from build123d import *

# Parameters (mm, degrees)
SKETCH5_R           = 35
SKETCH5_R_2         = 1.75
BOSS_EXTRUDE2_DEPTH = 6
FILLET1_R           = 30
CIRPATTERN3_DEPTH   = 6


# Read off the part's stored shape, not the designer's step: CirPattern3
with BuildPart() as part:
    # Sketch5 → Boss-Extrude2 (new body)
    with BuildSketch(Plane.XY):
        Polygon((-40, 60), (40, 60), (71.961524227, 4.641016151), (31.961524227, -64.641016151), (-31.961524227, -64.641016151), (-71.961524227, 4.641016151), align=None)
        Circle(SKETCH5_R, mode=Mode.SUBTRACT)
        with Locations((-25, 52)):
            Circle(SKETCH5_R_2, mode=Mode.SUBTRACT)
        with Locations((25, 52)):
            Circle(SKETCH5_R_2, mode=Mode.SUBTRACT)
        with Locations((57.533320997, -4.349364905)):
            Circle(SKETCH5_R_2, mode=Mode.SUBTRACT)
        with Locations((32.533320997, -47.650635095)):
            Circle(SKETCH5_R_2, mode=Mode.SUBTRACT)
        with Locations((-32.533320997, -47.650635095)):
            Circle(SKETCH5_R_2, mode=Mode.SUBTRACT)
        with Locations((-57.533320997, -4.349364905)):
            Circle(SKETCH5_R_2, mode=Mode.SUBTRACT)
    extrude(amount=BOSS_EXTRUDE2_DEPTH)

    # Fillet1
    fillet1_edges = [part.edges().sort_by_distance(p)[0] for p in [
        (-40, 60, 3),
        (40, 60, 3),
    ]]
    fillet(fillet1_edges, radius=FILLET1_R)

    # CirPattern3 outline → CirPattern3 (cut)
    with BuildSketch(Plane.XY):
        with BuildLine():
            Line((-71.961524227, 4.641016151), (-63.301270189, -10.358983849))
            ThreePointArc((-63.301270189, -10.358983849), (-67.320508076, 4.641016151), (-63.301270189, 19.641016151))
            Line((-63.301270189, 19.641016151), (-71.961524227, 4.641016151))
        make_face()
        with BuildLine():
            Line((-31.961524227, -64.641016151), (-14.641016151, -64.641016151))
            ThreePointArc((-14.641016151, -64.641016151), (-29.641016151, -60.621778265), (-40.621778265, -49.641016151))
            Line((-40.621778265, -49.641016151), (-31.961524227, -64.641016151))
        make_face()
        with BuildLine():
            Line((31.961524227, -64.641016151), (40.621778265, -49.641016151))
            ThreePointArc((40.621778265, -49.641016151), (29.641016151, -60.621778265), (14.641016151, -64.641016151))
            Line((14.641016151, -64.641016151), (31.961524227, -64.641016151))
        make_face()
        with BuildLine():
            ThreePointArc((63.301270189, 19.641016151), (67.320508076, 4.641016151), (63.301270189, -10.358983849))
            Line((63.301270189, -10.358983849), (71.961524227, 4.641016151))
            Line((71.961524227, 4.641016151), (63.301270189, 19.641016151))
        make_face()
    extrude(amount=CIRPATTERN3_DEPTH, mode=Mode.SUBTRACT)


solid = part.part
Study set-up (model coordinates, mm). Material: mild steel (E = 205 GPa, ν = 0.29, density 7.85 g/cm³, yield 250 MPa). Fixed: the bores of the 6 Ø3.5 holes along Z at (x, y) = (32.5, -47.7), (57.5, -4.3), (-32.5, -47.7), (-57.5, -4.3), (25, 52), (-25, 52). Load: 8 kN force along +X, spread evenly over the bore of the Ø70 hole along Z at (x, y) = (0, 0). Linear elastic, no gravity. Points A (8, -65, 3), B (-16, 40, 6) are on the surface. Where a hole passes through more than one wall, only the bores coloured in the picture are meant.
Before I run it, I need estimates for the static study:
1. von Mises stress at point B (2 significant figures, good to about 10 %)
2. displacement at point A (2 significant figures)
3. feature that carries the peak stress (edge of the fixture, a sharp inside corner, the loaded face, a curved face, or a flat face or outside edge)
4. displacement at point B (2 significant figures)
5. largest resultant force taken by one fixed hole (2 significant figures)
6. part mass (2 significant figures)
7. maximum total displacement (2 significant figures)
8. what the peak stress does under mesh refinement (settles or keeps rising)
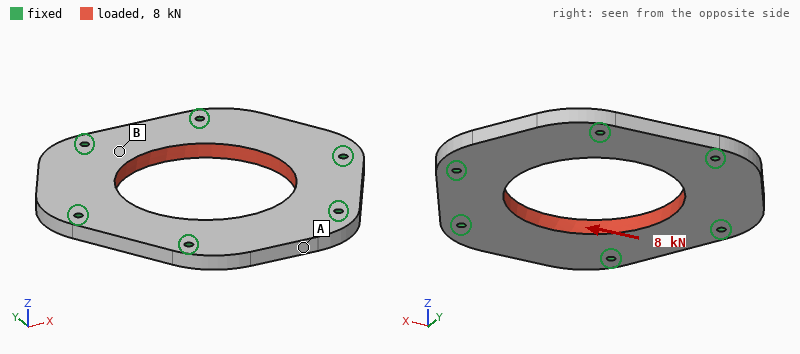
8.5 MPa
0.49 µm
edge of the fixture
1.2 µm
1.7 kN
430 g
2.5 µm
keeps rising
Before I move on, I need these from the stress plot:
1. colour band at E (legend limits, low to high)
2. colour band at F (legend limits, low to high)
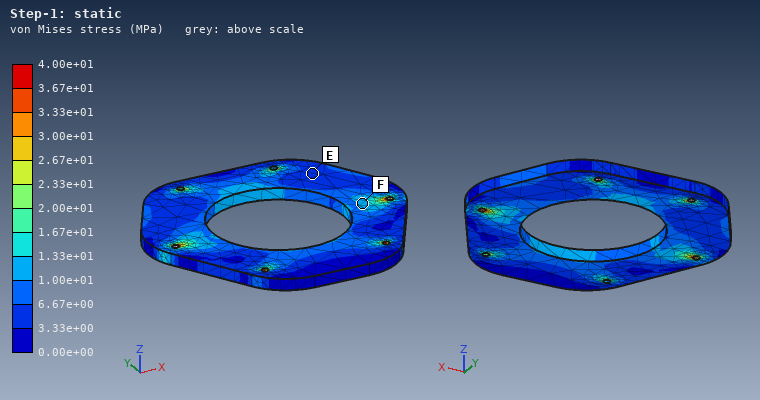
3.33e+00 to 6.67e+00 MPa
1.00e+01 to 1.33e+01 MPa
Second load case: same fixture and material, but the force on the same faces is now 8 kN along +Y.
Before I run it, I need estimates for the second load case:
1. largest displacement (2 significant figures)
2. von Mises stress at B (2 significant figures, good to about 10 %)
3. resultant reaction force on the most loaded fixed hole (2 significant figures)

2.7 µm
9.1 MPa
1.6 kN
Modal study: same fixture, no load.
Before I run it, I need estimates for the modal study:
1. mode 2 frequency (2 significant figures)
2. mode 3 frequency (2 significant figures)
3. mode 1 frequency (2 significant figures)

6000 Hz
6000 Hz
5900 Hz
